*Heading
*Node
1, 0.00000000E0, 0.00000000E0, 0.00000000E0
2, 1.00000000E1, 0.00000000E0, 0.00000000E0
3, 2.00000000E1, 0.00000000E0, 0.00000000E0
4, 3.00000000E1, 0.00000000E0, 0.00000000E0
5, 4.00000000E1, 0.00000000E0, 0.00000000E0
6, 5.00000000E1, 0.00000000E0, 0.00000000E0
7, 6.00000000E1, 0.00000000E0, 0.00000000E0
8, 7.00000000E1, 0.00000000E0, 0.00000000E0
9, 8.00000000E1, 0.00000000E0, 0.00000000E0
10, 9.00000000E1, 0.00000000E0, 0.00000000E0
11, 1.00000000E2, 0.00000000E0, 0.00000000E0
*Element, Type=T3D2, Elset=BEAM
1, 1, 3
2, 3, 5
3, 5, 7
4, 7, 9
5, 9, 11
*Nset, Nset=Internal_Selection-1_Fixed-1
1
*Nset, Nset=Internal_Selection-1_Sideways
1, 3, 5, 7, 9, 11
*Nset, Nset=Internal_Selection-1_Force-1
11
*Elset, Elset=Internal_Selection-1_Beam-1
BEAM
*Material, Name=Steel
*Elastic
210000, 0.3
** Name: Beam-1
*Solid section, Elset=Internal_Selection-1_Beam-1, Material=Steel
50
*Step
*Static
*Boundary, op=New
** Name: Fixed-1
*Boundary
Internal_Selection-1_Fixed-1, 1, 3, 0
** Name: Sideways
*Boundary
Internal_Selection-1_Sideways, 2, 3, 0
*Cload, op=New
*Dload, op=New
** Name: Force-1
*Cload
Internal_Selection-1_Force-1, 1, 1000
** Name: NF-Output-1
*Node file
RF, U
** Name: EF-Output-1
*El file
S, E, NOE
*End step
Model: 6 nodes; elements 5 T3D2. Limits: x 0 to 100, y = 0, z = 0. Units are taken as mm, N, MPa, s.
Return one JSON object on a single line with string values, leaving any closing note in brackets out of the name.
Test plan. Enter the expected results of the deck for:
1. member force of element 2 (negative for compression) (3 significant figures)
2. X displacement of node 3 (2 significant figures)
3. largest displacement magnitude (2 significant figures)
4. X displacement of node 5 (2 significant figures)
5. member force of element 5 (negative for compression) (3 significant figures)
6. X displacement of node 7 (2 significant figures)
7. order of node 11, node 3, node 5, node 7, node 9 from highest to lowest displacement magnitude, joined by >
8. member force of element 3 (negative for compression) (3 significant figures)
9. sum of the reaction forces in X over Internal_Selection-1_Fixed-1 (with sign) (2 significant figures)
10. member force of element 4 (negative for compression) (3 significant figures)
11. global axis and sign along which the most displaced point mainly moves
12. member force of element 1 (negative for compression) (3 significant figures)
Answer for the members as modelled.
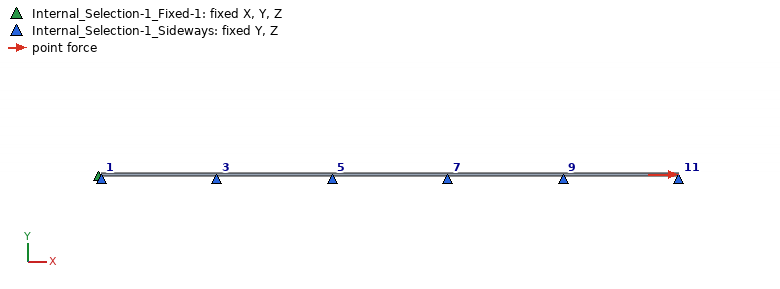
{"member force of element 2 (negative for compression)": "1000 N", "X displacement of node 3": "0.0019 mm", "largest displacement magnitude": "0.0095 mm", "X displacement of node 5": "0.0038 mm", "member force of element 5 (negative for compression)": "1000 N", "X displacement of node 7": "0.0057 mm", "order of node 11, node 3, node 5, node 7, node 9 from highest to lowest displacement magnitude, joined by >": "node 11 > node 9 > node 7 > node 5 > node 3", "member force of element 3 (negative for compression)": "1000 N", "sum of the reaction forces in X over Internal_Selection-1_Fixed-1 (with sign)": "-1000 N", "member force of element 4 (negative for compression)": "1000 N", "global axis and sign along which the most displaced point mainly moves": "+X", "member force of element 1 (negative for compression)": "1000 N"}
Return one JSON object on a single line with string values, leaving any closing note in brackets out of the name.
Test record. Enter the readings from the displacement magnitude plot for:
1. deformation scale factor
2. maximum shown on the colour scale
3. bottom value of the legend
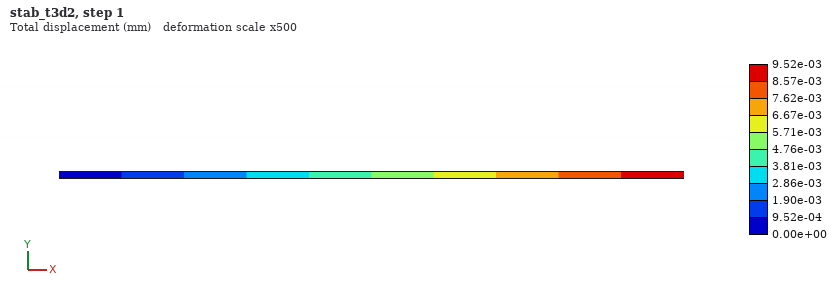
{"deformation scale factor": "500", "maximum shown on the colour scale": "9.52e-03 mm", "bottom value of the legend": "0.00e+00 mm"}
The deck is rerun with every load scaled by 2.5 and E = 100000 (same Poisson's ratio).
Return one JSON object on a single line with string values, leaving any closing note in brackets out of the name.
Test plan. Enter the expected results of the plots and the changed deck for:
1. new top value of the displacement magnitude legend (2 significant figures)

{"new top value of the displacement magnitude legend": "0.050 mm"}
